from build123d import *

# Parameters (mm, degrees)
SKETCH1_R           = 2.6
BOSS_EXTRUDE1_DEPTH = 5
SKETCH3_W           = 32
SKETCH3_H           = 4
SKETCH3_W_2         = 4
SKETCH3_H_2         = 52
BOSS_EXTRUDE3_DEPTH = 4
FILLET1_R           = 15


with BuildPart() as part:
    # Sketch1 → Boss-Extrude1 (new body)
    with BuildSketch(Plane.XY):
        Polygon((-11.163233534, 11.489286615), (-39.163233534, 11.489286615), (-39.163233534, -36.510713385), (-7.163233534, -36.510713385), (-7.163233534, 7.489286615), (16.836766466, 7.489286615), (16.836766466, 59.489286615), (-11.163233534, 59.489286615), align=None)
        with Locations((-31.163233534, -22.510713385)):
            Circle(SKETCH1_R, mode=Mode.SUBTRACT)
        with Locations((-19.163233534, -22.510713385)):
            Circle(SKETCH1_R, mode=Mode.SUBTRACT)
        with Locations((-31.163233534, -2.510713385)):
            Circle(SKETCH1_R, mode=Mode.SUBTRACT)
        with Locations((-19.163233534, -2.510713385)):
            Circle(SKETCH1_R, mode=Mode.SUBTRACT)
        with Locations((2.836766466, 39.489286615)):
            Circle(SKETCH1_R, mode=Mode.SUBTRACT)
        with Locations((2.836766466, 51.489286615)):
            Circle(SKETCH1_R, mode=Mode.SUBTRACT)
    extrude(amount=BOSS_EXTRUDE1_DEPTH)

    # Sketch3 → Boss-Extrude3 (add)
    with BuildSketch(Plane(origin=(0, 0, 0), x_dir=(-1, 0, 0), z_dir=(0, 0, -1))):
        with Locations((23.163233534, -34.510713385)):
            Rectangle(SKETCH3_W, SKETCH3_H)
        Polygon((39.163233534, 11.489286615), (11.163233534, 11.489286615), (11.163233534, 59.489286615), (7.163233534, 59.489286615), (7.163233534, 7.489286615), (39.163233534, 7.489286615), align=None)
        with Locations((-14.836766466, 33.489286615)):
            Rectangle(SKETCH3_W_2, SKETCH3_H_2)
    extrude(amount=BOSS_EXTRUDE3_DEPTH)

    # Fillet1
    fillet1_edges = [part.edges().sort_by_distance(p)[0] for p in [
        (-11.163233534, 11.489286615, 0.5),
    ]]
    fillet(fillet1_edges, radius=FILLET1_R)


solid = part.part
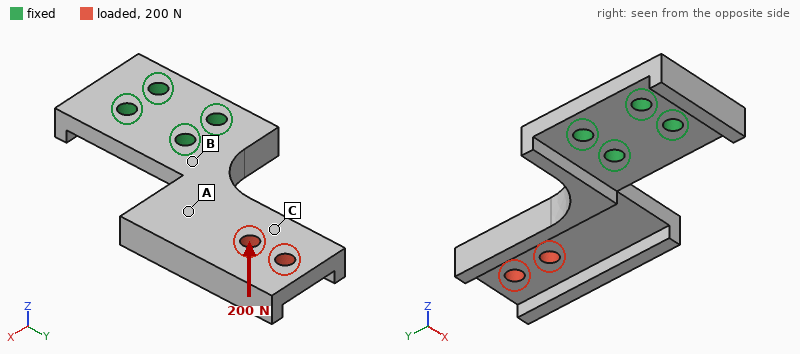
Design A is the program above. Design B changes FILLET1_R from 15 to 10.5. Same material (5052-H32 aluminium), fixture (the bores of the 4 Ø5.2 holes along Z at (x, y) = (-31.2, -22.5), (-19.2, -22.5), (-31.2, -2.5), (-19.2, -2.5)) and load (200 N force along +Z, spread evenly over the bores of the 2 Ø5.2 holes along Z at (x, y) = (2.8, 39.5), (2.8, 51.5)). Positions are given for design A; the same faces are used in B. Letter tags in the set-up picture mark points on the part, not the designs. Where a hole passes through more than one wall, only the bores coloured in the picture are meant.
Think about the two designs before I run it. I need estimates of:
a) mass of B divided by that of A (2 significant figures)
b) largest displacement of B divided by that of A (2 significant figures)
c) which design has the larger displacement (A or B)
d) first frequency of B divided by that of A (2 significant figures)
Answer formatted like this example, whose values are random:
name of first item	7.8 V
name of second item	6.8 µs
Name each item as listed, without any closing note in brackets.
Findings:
mass of B divided by that of A	0.99
largest displacement of B divided by that of A	1.1
which design has the larger displacement	B
first frequency of B divided by that of A	0.95
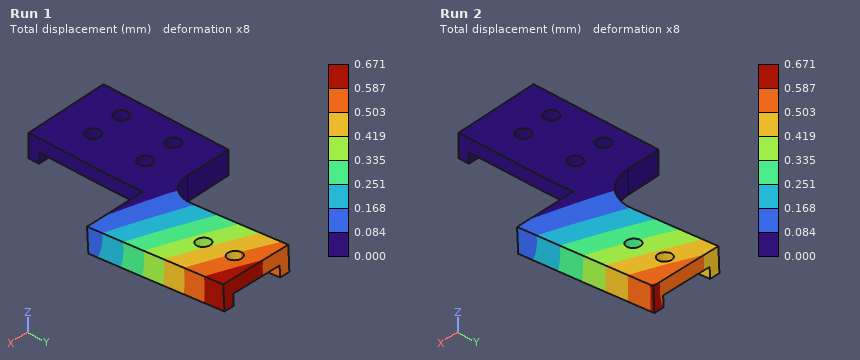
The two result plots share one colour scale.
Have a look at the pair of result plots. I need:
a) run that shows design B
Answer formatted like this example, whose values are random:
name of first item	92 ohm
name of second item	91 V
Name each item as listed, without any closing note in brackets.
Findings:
run that shows design B	Run 1
